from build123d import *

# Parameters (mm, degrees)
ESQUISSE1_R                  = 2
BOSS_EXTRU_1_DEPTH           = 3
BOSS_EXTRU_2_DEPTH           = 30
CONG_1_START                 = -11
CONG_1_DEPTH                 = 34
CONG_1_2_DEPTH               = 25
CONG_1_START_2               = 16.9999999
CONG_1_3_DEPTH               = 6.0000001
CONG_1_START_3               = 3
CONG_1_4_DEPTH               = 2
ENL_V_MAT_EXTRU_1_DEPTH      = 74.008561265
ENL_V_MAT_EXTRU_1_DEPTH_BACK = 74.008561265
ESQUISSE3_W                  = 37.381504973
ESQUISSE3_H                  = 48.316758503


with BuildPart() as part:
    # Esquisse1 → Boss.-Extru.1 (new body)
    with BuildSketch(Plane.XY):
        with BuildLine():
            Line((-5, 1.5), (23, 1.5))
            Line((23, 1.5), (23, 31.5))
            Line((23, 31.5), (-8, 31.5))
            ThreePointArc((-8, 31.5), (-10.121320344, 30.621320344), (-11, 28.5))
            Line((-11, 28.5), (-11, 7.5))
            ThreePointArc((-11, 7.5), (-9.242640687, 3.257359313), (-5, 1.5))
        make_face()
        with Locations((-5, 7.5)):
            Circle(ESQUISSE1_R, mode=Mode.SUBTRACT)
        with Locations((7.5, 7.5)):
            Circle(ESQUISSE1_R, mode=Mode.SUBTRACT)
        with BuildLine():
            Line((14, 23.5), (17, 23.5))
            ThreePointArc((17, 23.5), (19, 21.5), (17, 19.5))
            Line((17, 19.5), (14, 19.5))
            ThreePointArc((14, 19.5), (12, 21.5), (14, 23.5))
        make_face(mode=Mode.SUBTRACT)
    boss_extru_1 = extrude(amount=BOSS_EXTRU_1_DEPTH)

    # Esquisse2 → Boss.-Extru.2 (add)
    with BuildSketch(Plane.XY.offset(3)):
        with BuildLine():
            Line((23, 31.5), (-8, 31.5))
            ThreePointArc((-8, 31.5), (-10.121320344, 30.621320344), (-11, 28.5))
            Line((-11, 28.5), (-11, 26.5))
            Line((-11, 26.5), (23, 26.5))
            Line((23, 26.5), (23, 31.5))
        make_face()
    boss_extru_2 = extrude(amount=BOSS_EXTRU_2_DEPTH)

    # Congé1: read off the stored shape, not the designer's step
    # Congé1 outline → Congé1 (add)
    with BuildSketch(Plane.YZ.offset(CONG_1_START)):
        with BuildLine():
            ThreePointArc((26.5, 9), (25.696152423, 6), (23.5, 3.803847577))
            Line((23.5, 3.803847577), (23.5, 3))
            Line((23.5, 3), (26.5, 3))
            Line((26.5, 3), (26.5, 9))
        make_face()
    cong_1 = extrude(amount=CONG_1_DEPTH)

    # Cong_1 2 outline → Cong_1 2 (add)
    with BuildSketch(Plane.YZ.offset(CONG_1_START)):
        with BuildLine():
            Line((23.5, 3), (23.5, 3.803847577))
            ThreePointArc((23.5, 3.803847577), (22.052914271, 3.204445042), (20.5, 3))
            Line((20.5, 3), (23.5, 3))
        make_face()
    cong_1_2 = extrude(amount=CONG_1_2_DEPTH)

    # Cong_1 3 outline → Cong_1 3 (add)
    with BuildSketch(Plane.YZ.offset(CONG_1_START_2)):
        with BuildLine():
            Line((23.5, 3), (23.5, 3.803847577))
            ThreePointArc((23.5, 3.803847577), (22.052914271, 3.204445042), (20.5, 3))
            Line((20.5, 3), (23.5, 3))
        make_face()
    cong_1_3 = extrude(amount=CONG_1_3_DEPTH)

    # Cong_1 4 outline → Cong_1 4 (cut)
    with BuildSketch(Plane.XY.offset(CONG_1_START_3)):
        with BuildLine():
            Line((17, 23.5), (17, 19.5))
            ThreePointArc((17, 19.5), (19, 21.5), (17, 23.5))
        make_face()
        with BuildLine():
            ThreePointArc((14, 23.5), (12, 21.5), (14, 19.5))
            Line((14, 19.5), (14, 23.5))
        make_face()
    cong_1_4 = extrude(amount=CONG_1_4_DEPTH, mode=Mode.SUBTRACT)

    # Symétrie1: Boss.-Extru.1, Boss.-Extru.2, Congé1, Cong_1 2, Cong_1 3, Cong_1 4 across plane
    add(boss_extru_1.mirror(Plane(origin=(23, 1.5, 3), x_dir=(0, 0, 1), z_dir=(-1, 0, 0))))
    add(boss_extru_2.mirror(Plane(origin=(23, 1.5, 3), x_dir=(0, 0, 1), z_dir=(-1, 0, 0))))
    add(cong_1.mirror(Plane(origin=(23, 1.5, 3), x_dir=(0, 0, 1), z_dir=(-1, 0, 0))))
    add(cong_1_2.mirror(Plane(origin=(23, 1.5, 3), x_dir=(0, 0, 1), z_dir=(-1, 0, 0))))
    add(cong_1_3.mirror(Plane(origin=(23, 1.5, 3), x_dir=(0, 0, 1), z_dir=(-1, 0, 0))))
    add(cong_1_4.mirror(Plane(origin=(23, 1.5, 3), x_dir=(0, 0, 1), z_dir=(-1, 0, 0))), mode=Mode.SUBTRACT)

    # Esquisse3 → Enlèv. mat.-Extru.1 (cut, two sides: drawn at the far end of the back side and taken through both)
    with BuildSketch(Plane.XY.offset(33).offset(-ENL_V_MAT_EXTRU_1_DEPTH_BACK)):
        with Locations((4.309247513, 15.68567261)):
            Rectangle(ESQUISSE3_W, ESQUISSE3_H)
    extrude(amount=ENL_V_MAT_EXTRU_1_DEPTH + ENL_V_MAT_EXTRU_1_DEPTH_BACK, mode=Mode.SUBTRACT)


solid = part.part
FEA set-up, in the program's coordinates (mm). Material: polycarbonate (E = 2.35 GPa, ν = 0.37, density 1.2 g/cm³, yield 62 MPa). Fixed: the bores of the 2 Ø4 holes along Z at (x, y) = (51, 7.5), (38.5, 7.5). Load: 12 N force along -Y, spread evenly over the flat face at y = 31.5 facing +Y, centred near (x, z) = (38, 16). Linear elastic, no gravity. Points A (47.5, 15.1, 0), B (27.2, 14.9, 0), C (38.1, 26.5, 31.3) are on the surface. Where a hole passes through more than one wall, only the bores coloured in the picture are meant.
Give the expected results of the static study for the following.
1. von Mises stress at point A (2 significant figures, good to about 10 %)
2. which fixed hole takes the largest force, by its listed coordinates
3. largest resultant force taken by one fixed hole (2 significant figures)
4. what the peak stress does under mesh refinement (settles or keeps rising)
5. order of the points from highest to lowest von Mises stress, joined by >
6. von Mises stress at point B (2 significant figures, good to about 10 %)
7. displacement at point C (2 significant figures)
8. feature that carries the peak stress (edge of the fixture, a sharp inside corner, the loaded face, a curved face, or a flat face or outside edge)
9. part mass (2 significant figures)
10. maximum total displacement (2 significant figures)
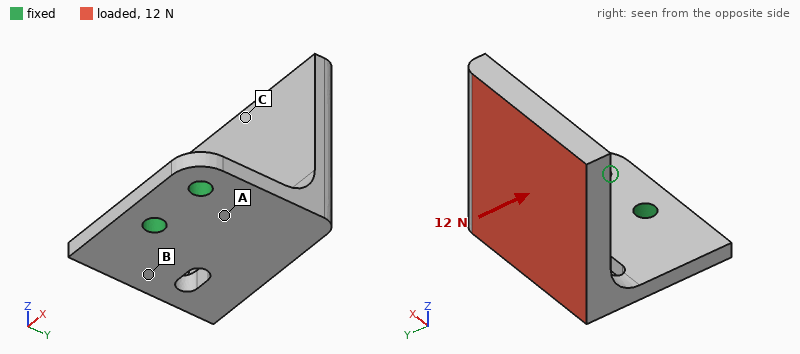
3.5 MPa
(38.5, 7.5)
11 N
keeps rising
A > B > C
2.4 MPa
0.57 mm
edge of the fixture
9.8 g
0.64 mm
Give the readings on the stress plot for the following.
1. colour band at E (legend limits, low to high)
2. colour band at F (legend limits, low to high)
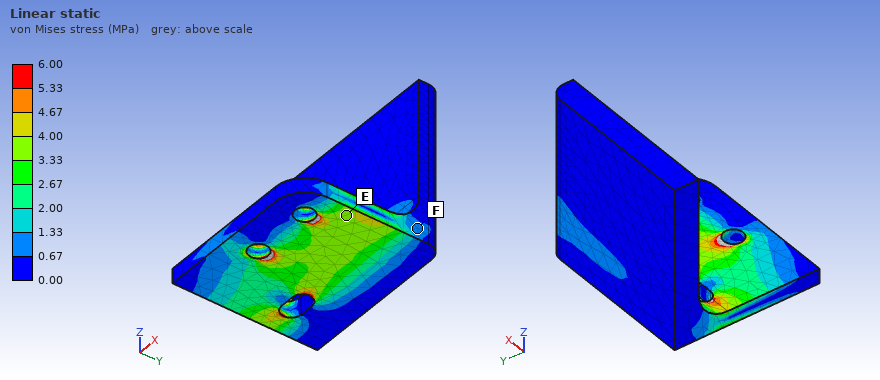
3.33 to 4.00 MPa
0.67 to 1.33 MPa
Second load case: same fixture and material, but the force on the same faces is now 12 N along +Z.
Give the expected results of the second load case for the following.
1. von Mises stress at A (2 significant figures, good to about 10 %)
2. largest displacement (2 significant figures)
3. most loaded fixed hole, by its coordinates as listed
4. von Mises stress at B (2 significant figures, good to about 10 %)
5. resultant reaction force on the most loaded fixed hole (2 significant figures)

3.9 MPa
0.65 mm
(38.5, 7.5)
2.6 MPa
9.9 N
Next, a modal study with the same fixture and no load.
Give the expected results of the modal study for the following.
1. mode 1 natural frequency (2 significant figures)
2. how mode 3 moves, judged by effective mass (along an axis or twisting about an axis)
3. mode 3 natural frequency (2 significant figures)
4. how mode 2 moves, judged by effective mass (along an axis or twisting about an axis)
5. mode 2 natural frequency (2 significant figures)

280 Hz
along Z
1200 Hz
along X
520 Hz
